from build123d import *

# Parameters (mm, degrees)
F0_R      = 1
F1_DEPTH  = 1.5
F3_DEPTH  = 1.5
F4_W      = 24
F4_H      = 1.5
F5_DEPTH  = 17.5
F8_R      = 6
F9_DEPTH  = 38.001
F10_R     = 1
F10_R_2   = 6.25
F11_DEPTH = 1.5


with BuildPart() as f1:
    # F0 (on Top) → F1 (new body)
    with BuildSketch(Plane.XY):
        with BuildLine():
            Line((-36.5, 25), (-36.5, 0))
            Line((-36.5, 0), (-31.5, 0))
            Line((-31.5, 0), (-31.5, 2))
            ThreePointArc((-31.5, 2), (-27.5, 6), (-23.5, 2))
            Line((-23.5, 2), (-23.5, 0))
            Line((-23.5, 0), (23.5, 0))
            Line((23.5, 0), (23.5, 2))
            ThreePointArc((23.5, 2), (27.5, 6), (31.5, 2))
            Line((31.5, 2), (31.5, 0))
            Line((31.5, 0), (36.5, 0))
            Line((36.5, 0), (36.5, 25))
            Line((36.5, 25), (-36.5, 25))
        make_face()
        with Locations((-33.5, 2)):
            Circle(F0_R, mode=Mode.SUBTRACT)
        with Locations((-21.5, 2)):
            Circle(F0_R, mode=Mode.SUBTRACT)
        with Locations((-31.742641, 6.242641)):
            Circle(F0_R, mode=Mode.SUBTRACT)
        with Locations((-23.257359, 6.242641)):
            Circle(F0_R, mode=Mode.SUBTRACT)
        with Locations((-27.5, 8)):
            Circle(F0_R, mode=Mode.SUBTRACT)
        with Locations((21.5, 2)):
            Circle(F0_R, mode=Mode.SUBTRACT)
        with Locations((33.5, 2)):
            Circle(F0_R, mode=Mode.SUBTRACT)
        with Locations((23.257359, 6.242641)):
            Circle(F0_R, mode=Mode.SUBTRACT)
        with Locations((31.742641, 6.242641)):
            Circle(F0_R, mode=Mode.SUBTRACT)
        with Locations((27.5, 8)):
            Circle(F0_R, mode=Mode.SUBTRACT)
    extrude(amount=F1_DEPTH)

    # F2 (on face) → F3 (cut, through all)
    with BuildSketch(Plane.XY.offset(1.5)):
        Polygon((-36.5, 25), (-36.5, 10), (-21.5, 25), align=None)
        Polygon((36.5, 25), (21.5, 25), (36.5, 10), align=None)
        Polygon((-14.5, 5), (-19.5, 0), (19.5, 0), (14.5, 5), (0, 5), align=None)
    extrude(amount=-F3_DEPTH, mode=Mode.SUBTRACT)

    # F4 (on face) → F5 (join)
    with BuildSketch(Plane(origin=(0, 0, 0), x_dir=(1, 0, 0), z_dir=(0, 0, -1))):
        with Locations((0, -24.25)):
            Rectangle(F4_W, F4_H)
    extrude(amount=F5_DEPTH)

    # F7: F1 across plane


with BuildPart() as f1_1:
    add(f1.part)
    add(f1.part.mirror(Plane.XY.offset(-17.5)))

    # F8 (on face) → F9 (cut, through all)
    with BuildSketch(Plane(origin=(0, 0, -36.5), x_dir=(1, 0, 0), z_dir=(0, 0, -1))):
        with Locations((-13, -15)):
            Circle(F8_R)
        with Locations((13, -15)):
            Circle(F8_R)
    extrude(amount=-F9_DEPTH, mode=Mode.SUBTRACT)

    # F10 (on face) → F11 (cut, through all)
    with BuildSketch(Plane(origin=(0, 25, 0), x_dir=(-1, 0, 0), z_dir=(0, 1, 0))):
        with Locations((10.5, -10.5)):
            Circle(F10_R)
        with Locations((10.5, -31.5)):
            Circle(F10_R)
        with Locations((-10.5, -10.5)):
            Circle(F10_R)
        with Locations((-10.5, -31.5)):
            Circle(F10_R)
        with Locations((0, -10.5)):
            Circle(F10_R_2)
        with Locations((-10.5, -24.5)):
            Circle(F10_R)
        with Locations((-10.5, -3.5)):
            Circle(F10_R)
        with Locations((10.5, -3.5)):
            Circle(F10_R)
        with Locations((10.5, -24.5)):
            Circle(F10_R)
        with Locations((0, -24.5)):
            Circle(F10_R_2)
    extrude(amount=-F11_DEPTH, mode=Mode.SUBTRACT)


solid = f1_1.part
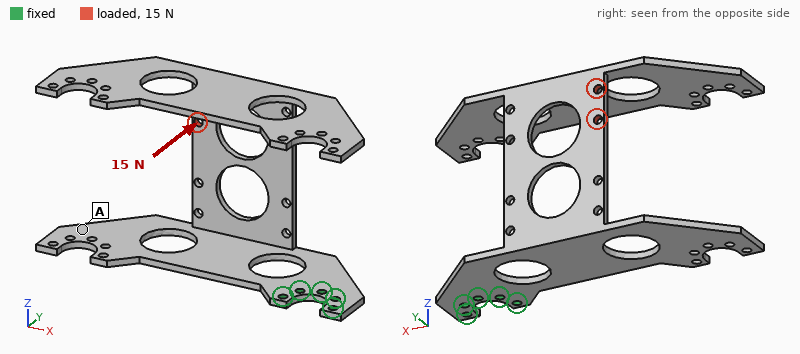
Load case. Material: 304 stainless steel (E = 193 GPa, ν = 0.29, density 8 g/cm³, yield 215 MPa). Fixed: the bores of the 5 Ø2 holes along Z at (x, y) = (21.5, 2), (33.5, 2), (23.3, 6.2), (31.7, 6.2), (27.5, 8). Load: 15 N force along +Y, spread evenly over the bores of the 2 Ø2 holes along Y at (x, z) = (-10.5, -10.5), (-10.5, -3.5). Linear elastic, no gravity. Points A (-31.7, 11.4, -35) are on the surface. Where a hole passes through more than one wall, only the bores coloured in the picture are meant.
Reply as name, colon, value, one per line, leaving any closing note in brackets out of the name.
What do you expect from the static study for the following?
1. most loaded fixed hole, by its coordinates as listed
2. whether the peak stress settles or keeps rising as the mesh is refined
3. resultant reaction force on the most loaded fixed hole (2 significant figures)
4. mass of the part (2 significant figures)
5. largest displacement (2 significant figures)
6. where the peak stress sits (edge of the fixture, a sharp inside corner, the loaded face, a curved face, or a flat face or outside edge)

most loaded fixed hole, by its coordinates as listed: (21.5, 2)
whether the peak stress settles or keeps rising as the mesh is refined: keeps rising
resultant reaction force on the most loaded fixed hole: 53 N
mass of the part: 33 g
largest displacement: 0.80 mm
where the peak stress sits: a sharp inside corner
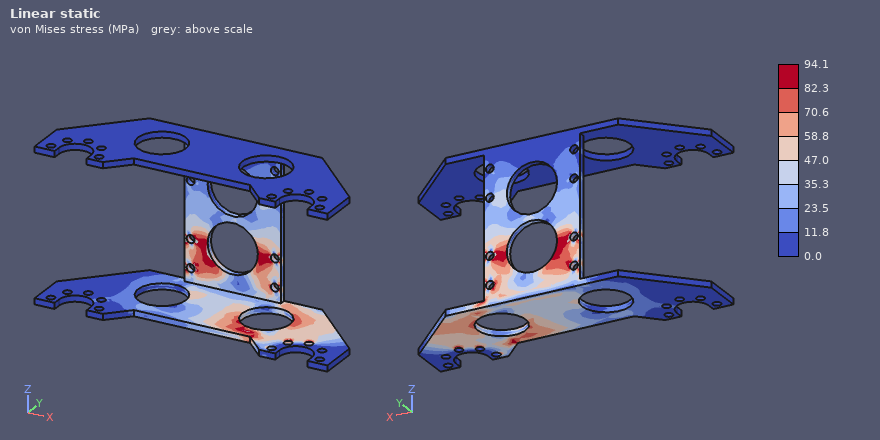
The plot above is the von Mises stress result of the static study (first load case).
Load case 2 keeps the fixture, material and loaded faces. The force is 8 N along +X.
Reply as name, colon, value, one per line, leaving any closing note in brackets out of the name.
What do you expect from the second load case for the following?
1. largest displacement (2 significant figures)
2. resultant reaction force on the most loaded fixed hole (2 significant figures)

largest displacement: 0.41 mm
resultant reaction force on the most loaded fixed hole: 19 N
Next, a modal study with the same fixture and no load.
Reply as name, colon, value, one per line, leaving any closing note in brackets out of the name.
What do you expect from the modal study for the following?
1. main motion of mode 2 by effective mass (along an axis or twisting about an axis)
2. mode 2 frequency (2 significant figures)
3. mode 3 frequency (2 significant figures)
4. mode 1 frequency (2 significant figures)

main motion of mode 2 by effective mass: along Y
mode 2 frequency: 180 Hz
mode 3 frequency: 360 Hz
mode 1 frequency: 140 Hz
